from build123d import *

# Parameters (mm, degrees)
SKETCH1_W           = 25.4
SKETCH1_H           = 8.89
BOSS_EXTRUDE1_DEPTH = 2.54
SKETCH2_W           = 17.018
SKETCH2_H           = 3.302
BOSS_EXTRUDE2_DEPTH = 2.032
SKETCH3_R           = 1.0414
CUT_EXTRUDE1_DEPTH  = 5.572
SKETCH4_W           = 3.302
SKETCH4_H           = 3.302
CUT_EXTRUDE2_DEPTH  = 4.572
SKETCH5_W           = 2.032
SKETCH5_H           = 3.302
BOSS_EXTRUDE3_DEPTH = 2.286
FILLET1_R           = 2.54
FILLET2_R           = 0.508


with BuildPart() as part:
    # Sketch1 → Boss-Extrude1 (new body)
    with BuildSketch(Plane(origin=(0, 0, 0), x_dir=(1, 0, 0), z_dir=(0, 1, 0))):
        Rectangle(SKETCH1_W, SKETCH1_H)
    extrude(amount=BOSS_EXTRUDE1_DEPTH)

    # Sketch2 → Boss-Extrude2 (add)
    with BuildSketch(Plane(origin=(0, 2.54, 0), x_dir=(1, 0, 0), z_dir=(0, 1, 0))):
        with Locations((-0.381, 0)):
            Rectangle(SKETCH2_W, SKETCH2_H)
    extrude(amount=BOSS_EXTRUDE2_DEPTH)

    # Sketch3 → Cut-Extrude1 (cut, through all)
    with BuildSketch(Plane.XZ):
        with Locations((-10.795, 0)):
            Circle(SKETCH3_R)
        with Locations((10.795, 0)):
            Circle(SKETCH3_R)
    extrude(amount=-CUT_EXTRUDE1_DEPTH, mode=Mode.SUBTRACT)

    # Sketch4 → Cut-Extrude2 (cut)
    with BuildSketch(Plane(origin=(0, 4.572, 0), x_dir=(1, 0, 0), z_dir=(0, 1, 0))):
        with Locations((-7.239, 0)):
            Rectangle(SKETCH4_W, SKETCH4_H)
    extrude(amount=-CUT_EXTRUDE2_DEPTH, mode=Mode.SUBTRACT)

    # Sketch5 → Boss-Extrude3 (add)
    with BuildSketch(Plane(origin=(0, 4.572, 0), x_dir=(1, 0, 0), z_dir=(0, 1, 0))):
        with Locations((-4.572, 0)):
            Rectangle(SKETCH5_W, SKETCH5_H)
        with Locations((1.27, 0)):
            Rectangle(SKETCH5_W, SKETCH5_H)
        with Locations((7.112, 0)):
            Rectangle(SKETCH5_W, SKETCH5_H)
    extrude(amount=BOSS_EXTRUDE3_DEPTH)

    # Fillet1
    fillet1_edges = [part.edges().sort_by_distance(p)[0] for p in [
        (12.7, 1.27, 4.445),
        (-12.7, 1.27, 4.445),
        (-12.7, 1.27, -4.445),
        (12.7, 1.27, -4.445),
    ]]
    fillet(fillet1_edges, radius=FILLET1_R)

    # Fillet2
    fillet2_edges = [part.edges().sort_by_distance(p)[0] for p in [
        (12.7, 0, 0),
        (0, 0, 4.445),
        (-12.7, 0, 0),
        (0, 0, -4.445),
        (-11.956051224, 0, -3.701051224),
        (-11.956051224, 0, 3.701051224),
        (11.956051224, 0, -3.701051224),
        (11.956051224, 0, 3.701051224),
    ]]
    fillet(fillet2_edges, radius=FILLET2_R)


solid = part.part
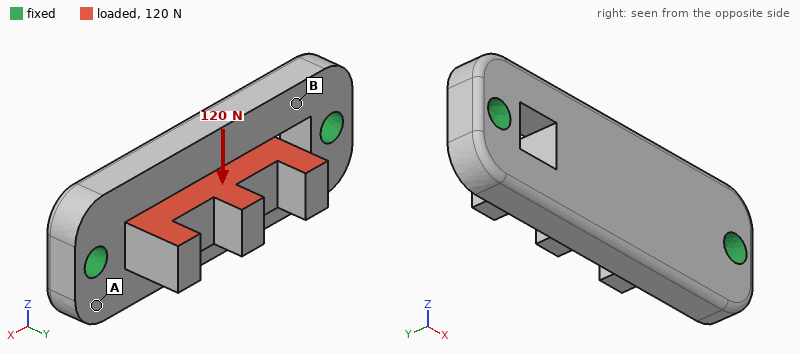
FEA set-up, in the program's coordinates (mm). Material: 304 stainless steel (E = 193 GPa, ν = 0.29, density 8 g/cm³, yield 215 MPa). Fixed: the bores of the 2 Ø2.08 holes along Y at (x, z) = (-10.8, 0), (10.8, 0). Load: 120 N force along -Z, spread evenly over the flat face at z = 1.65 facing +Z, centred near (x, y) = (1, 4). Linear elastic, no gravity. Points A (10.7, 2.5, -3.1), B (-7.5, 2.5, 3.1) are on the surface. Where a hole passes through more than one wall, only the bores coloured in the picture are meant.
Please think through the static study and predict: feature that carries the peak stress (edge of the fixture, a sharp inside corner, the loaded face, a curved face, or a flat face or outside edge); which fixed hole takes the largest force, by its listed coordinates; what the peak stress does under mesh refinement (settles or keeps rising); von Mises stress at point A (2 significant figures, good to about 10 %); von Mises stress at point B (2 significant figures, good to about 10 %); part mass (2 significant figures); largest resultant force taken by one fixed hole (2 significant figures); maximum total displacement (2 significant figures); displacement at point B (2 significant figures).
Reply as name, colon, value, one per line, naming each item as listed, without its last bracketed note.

feature that carries the peak stress: edge of the fixture
which fixed hole takes the largest force, by its listed coordinates: (10.8, 0)
what the peak stress does under mesh refinement: keeps rising
von Mises stress at point A: 7.5 MPa
von Mises stress at point B: 20 MPa
part mass: 5.2 g
largest resultant force taken by one fixed hole: 73 N
maximum total displacement: 3.3 µm
displacement at point B: 0.89 µm
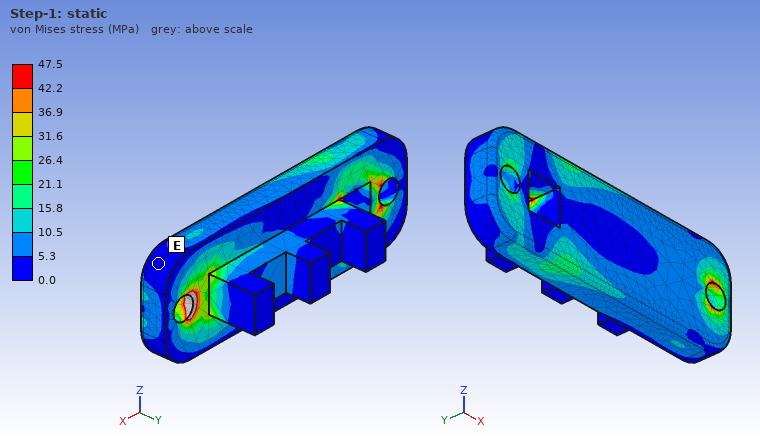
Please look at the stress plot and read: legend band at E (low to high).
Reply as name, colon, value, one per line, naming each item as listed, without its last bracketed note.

legend band at E: 0.0 to 5.3 MPa
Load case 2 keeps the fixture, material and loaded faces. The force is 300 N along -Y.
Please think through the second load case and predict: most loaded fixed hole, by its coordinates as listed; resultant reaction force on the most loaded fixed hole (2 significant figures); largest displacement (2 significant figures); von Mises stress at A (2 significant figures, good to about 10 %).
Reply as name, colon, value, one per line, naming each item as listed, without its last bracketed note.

most loaded fixed hole, by its coordinates as listed: (10.8, 0)
resultant reaction force on the most loaded fixed hole: 180 N
largest displacement: 6.8 µm
von Mises stress at A: 14 MPa
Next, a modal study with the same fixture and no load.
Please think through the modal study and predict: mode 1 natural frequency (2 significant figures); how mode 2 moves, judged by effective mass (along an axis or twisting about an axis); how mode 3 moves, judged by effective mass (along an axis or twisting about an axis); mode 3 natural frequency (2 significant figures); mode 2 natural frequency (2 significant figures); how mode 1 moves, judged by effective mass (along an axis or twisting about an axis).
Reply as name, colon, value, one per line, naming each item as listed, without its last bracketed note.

mode 1 natural frequency: 23 kHz
how mode 2 moves, judged by effective mass: along Z
how mode 3 moves, judged by effective mass: along Z
mode 3 natural frequency: 35 kHz
mode 2 natural frequency: 26 kHz
how mode 1 moves, judged by effective mass: along Y
